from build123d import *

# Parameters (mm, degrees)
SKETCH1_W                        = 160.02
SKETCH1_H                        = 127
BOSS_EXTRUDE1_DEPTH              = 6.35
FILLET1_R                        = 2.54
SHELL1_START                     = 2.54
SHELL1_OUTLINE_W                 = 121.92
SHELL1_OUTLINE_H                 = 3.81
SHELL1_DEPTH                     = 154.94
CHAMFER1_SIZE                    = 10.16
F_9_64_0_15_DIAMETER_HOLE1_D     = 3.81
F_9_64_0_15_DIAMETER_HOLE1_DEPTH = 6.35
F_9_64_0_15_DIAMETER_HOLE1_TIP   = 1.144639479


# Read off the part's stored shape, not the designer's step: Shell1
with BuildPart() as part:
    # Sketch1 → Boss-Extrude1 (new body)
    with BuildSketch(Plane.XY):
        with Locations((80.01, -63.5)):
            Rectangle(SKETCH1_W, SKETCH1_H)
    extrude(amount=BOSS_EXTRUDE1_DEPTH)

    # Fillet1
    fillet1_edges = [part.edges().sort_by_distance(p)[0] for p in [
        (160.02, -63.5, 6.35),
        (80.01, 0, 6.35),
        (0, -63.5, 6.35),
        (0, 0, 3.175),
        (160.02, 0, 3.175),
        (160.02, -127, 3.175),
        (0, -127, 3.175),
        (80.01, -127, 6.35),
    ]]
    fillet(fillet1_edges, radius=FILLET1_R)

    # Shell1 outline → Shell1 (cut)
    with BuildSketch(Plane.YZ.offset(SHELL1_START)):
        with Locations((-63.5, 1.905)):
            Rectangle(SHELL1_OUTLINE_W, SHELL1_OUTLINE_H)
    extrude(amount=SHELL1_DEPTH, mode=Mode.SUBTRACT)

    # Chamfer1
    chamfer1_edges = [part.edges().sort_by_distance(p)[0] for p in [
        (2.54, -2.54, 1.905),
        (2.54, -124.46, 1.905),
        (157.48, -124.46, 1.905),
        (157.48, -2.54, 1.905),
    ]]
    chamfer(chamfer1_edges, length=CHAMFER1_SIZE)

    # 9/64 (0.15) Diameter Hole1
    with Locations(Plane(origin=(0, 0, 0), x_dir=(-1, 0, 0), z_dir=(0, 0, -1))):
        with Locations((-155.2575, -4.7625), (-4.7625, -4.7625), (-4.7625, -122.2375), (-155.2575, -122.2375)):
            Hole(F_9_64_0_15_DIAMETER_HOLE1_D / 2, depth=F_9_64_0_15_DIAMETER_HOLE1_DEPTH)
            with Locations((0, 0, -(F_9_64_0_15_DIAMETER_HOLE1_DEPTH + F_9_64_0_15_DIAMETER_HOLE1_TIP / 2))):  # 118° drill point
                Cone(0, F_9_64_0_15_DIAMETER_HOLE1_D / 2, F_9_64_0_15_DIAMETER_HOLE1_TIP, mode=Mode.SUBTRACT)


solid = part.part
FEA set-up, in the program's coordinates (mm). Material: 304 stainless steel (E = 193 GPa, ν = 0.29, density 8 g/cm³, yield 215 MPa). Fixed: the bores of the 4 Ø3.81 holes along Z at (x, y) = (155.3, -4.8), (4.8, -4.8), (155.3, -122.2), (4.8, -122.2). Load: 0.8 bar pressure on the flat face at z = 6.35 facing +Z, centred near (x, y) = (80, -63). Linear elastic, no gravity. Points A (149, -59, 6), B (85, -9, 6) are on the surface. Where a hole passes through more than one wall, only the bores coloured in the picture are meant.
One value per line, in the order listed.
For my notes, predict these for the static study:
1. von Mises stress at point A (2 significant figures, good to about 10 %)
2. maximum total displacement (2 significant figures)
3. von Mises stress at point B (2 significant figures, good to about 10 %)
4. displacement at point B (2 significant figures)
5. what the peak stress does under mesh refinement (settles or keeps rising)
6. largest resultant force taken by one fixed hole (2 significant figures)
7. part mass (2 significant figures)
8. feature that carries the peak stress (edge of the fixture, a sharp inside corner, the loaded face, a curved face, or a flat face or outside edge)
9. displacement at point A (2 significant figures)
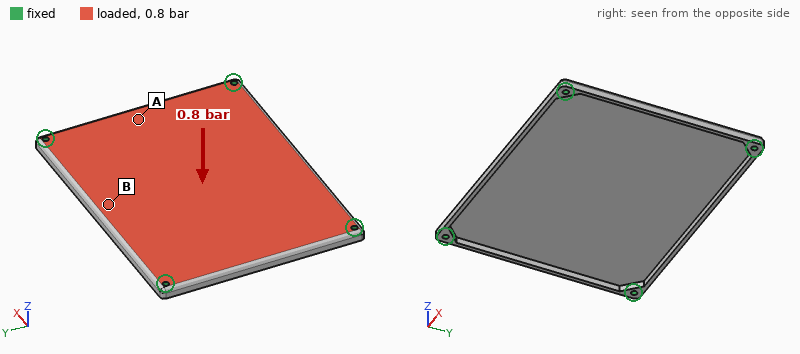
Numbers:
32 MPa
0.48 mm
47 MPa
0.24 mm
keeps rising
670 N
450 g
edge of the fixture
0.14 mm
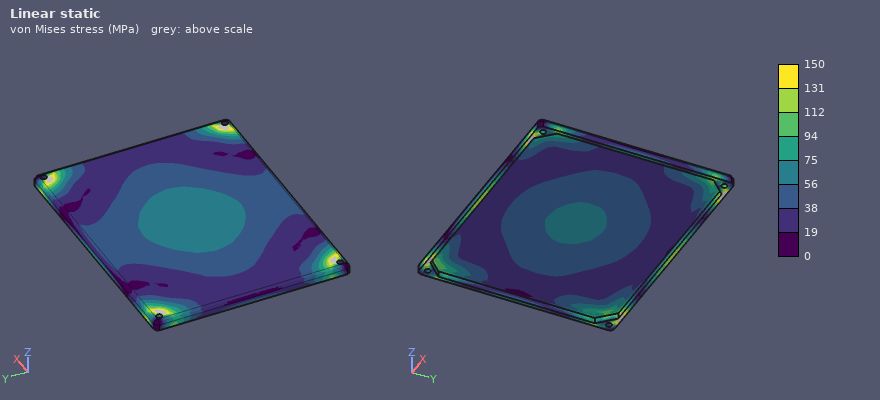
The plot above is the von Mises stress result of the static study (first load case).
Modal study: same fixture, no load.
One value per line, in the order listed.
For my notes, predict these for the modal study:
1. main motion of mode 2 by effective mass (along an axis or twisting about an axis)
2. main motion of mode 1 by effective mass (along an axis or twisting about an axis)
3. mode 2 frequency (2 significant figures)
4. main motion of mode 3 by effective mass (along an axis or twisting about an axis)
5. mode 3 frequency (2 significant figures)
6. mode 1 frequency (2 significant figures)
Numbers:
twisting about X
along Z
1100 Hz
twisting about Y
1200 Hz
560 Hz
